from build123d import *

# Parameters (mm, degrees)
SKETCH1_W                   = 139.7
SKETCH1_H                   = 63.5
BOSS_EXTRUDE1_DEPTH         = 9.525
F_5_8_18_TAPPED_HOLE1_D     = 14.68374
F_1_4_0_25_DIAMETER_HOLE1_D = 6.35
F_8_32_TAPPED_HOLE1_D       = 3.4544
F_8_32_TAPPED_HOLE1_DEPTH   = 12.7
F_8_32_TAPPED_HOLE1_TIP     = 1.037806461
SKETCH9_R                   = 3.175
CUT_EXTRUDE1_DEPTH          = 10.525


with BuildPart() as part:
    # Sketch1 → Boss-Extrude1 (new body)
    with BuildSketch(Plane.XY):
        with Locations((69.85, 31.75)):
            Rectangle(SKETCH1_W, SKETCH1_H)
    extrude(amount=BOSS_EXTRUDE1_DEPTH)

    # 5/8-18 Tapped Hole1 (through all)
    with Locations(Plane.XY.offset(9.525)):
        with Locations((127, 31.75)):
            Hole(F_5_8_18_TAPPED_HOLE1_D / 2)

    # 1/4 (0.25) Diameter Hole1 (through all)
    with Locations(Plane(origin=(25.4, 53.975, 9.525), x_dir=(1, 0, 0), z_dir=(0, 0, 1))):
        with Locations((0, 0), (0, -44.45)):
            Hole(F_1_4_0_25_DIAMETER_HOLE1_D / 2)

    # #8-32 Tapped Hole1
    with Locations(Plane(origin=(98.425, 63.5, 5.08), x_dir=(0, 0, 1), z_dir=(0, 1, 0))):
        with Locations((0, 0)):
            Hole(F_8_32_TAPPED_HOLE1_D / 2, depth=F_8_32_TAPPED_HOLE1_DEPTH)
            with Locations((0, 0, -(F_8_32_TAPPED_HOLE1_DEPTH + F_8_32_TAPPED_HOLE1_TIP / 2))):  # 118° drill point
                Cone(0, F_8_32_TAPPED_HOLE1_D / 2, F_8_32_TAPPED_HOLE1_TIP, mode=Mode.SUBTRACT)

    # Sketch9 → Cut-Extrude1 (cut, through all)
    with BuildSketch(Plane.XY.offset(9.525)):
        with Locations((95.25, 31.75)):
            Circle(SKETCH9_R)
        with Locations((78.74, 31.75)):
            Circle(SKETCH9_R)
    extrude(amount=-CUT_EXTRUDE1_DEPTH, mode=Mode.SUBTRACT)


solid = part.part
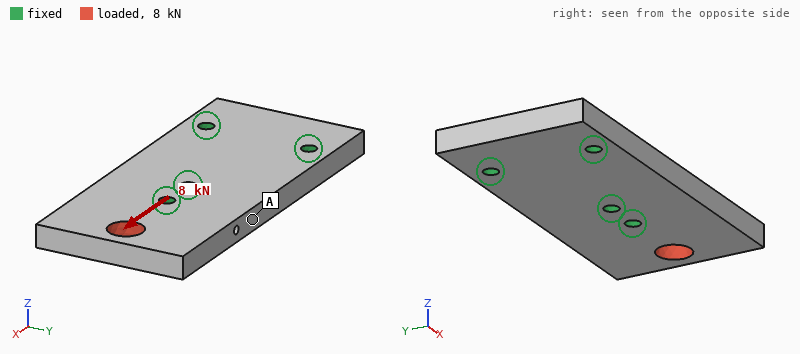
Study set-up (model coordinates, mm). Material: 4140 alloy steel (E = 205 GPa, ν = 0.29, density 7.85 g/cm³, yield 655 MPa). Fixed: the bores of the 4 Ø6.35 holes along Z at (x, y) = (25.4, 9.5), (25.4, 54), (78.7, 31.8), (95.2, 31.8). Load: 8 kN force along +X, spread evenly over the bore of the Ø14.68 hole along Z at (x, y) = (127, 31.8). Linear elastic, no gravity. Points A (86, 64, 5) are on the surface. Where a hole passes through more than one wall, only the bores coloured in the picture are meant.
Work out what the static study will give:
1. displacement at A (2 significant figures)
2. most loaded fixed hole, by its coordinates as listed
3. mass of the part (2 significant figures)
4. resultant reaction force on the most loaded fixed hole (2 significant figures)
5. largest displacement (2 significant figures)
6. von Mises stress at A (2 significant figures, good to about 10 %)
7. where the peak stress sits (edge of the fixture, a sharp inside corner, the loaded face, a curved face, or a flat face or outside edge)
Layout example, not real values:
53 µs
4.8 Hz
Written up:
1.4 µm
(95.2, 31.8)
640 g
4.9 kN
7.8 µm
7.1 MPa
the loaded face
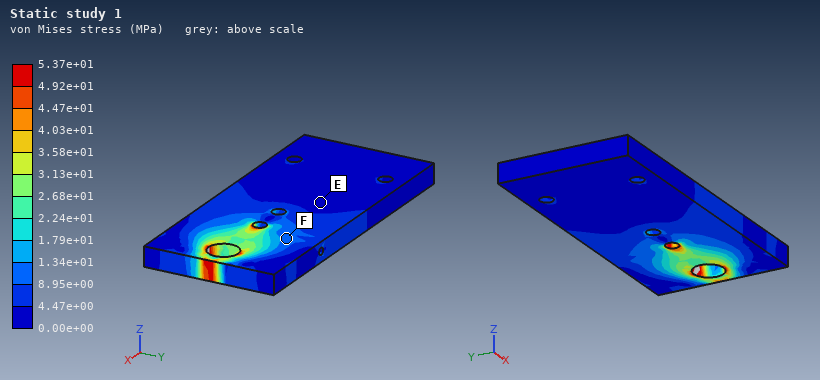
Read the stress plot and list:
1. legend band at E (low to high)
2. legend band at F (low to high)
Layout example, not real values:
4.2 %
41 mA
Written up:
0.00e+00 to 4.47e+00 MPa
8.95e+00 to 1.34e+01 MPa
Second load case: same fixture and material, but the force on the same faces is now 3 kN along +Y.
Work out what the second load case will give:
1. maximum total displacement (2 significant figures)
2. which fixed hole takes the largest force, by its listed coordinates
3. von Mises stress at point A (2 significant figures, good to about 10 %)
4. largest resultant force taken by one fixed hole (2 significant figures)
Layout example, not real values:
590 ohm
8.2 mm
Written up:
9.7 µm
(95.2, 31.8)
14 MPa
4.3 kN
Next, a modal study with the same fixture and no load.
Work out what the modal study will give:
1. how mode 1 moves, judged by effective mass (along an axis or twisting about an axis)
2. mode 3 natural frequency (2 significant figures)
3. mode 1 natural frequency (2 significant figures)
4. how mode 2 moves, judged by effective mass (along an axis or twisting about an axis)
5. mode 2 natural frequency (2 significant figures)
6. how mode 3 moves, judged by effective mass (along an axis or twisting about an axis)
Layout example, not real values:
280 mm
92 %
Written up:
along Z
8700 Hz
3400 Hz
twisting about X
4200 Hz
along Z
